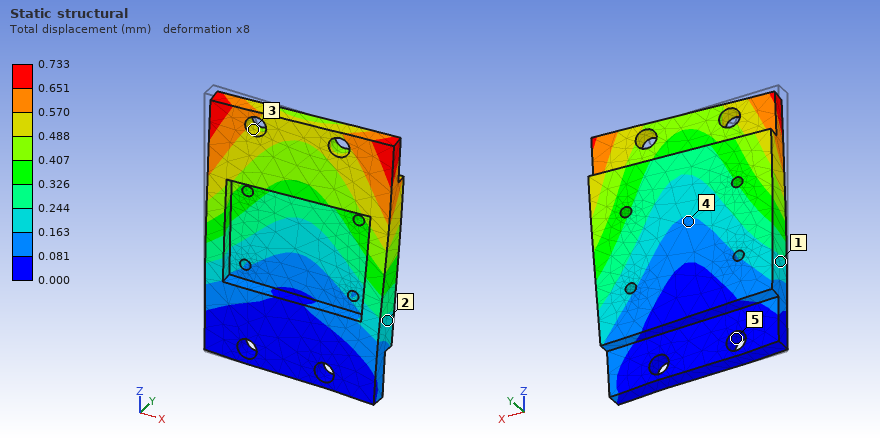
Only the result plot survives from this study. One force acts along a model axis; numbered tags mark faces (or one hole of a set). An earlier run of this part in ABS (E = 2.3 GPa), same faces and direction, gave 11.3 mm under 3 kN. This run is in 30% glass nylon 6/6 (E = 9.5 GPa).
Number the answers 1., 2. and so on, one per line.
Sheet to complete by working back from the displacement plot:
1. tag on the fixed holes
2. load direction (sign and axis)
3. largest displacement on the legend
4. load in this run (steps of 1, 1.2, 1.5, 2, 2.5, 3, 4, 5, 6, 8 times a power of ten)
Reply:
1. 5
2. +X
3. 0.733 mm
4. 800 N
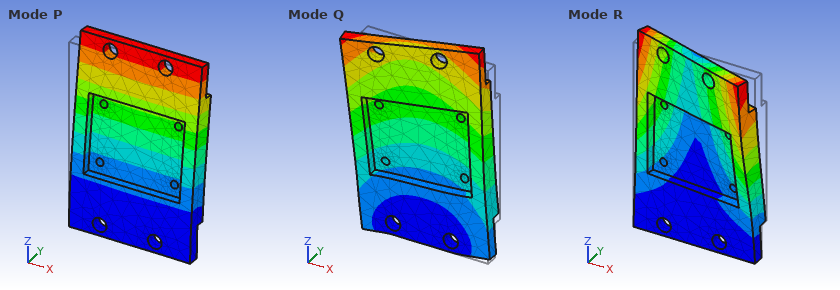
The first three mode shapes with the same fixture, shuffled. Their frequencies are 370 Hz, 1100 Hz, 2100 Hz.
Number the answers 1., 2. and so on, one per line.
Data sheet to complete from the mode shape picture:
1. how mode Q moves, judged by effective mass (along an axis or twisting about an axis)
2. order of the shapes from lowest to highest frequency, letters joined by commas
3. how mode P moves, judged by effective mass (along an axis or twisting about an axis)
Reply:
1. along X
2. P, R, Q
3. along Y
